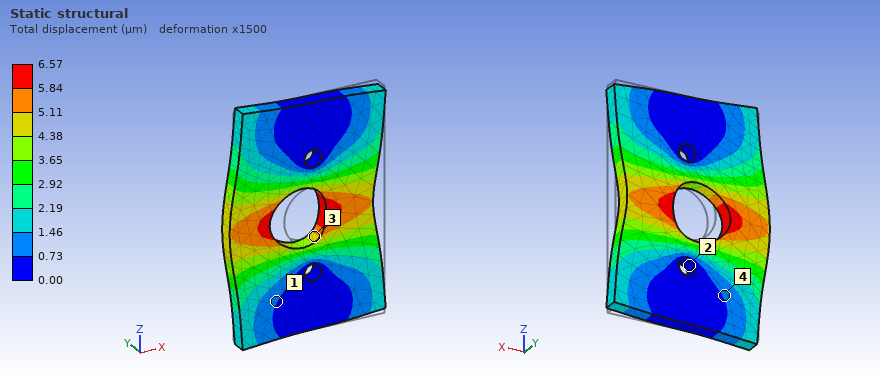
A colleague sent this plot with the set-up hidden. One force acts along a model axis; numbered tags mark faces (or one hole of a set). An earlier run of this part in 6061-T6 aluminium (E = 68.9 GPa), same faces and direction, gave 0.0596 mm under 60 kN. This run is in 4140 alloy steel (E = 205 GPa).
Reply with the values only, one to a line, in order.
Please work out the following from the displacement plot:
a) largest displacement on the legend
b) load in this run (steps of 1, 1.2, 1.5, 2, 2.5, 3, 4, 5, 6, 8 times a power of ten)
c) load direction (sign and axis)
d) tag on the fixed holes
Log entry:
6.57 µm
20 kN
-X
2
